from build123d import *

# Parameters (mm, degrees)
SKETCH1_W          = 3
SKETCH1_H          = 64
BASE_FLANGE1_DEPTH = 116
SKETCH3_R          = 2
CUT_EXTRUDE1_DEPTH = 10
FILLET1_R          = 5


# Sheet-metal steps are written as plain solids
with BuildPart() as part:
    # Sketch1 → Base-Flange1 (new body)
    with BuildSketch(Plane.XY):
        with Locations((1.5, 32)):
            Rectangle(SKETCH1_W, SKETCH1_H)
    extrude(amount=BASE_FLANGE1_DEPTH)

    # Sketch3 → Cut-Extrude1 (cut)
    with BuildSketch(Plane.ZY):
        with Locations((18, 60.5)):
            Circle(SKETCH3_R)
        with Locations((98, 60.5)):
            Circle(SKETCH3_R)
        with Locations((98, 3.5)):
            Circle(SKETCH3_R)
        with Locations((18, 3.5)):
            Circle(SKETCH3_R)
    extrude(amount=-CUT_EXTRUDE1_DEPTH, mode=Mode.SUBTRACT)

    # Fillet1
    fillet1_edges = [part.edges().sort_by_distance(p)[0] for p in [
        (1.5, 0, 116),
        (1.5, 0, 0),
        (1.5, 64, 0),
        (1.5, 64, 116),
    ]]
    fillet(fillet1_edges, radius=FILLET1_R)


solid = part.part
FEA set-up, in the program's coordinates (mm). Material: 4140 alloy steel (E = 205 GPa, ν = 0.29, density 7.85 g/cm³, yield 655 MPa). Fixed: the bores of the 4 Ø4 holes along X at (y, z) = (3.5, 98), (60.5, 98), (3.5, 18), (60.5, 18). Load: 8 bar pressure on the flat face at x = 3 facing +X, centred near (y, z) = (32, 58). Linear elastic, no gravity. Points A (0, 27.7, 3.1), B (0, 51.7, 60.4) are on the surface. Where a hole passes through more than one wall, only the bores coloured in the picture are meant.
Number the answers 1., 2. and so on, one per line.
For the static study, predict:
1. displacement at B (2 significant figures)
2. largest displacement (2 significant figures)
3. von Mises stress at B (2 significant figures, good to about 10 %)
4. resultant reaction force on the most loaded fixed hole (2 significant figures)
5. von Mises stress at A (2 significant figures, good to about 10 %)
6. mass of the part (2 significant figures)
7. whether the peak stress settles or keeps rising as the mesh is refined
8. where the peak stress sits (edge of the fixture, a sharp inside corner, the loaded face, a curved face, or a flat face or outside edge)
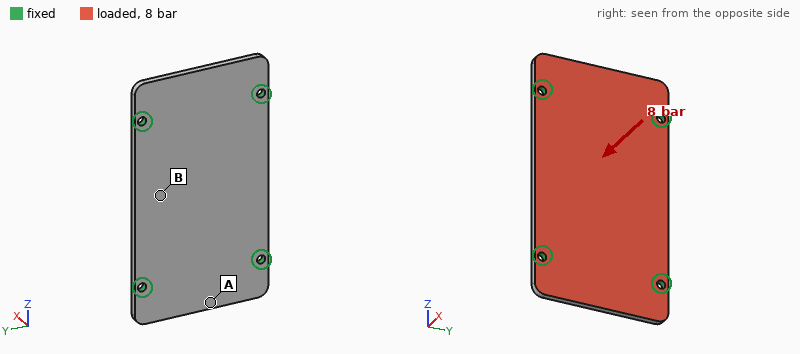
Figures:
1. 0.26 mm
2. 0.28 mm
3. 150 MPa
4. 1.5 kN
5. 69 MPa
6. 170 g
7. keeps rising
8. edge of the fixture
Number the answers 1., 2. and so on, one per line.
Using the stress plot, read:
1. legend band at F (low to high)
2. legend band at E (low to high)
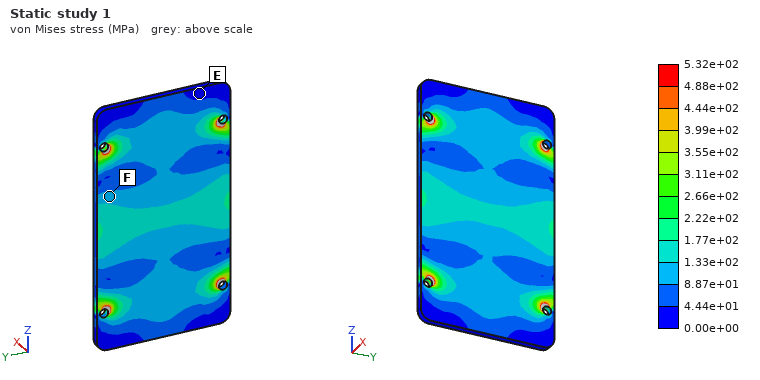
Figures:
1. 8.87e+01 to 1.33e+02 MPa
2. 0.00e+00 to 4.44e+01 MPa
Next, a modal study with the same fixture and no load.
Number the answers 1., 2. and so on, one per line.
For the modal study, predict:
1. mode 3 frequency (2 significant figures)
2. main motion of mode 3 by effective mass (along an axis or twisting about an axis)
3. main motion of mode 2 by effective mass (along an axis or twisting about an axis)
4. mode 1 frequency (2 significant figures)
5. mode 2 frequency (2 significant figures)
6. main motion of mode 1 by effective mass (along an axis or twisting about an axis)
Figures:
1. 3900 Hz
2. along X
3. twisting about Z
4. 2000 Hz
5. 3200 Hz
6. along X
